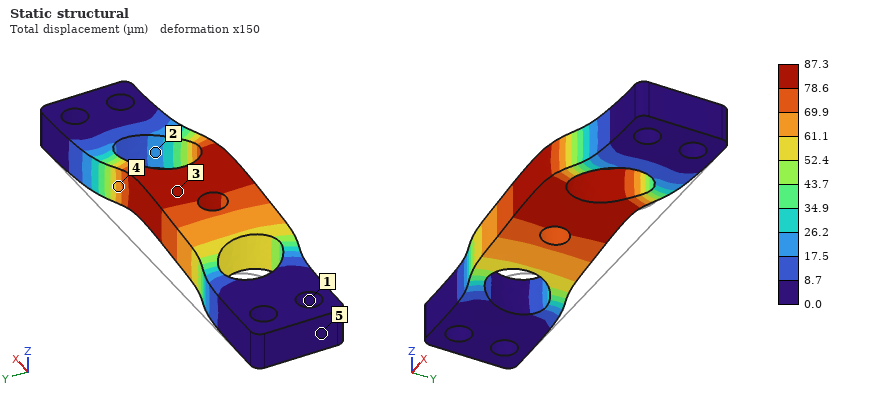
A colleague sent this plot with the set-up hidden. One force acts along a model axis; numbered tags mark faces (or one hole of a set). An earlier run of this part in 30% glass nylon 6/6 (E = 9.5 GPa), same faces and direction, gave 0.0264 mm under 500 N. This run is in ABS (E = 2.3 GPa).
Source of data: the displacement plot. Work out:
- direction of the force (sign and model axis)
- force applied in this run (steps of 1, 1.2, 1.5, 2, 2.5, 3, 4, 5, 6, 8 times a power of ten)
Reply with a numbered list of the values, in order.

1. -Y
2. 400 N
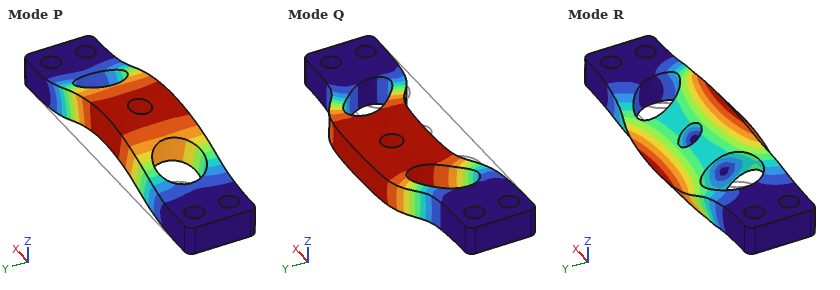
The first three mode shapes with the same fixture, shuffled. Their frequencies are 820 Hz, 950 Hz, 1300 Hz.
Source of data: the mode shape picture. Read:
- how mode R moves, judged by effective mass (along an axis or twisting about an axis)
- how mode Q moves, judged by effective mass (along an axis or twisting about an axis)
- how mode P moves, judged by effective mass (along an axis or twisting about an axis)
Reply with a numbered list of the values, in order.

1. twisting about X
2. along Y
3. along Z
